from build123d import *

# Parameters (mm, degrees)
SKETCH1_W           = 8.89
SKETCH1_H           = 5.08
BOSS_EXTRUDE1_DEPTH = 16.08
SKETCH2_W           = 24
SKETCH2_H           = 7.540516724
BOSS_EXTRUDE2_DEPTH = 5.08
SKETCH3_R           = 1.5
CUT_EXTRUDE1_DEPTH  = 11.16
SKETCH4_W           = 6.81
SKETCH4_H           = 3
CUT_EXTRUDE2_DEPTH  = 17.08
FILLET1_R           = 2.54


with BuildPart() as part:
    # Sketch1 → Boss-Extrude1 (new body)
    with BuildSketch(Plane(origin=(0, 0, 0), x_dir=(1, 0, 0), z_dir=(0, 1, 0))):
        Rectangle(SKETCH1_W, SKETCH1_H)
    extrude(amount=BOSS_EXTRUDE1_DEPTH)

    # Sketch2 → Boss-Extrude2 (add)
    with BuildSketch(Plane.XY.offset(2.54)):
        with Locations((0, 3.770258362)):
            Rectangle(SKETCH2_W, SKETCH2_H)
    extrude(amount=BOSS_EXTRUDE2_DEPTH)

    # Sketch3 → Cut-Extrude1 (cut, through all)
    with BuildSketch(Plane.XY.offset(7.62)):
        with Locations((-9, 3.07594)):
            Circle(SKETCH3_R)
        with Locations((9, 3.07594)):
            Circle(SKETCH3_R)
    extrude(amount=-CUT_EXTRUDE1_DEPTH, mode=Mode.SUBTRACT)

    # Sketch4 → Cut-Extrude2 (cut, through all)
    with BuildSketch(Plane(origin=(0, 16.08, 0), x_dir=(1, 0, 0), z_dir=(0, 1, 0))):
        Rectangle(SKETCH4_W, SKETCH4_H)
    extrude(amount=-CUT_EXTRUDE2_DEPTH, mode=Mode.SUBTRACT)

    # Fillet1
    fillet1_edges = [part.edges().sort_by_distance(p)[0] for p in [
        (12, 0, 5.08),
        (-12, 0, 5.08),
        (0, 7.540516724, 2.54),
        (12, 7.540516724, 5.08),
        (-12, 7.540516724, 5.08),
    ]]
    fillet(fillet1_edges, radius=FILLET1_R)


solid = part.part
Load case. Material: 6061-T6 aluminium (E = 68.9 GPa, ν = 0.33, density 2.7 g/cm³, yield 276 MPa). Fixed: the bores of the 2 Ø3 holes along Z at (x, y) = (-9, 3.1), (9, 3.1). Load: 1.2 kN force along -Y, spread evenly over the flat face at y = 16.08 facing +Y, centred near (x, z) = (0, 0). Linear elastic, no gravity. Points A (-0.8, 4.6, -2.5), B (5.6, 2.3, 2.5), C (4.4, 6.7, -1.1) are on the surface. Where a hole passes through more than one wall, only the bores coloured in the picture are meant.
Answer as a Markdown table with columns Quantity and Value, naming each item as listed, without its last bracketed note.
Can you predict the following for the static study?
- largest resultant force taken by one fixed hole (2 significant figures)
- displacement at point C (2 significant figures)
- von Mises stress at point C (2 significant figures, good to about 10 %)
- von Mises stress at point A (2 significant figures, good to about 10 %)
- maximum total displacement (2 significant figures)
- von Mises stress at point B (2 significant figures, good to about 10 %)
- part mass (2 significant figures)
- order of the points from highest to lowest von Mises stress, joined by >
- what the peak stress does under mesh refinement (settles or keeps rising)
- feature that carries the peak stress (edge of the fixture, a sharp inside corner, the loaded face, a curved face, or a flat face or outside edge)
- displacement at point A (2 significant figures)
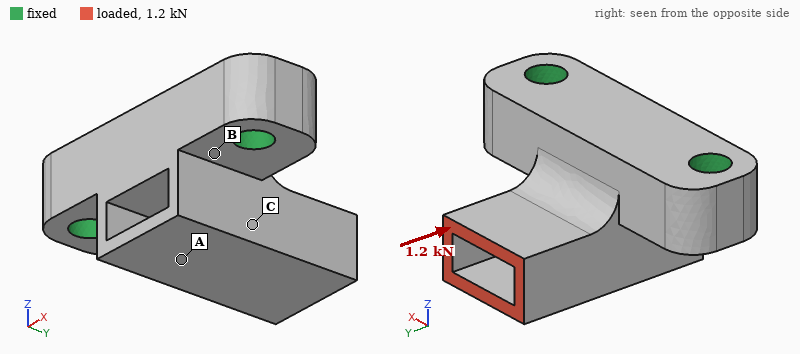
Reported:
| Quantity | Value |
|---|---|
| largest resultant force taken by one fixed hole | 620 N |
| displacement at point C | 35 µm |
| von Mises stress at point C | 65 MPa |
| von Mises stress at point A | 25 MPa |
| maximum total displacement | 76 µm |
| von Mises stress at point B | 130 MPa |
| part mass | 3.3 g |
| order of the points from highest to lowest von Mises stress, joined by > | B > C > A |
| what the peak stress does under mesh refinement | keeps rising |
| feature that carries the peak stress | edge of the fixture |
| displacement at point A | 40 µm |
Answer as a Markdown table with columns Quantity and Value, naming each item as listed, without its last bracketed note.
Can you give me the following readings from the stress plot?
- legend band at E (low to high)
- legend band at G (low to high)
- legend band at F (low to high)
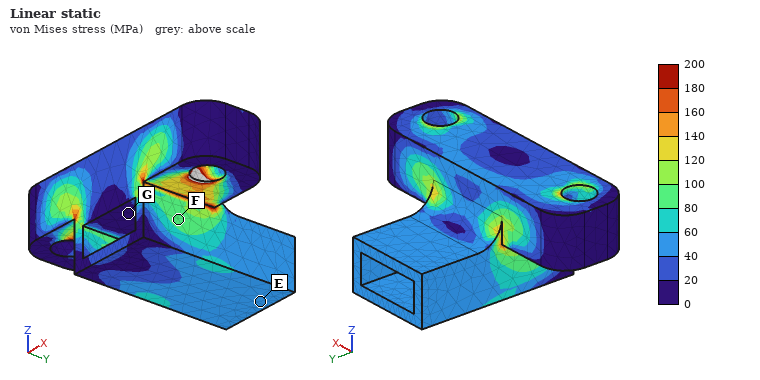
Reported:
| Quantity | Value |
|---|---|
| legend band at E | 40 to 60 MPa |
| legend band at G | 0 to 20 MPa |
| legend band at F | 80 to 100 MPa |
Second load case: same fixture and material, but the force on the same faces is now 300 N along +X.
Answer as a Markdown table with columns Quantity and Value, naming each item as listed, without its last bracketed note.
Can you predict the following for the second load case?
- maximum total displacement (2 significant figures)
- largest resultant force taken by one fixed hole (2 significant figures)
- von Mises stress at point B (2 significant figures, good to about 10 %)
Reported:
| Quantity | Value |
|---|---|
| maximum total displacement | 34 µm |
| largest resultant force taken by one fixed hole | 300 N |
| von Mises stress at point B | 22 MPa |
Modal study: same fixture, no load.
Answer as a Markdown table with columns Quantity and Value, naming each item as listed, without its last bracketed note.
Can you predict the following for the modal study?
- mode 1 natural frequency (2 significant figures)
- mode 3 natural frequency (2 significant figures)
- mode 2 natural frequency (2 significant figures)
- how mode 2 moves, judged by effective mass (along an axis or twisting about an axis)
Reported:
| Quantity | Value |
|---|---|
| mode 1 natural frequency | 19 kHz |
| mode 3 natural frequency | 35 kHz |
| mode 2 natural frequency | 27 kHz |
| how mode 2 moves, judged by effective mass | along X |
